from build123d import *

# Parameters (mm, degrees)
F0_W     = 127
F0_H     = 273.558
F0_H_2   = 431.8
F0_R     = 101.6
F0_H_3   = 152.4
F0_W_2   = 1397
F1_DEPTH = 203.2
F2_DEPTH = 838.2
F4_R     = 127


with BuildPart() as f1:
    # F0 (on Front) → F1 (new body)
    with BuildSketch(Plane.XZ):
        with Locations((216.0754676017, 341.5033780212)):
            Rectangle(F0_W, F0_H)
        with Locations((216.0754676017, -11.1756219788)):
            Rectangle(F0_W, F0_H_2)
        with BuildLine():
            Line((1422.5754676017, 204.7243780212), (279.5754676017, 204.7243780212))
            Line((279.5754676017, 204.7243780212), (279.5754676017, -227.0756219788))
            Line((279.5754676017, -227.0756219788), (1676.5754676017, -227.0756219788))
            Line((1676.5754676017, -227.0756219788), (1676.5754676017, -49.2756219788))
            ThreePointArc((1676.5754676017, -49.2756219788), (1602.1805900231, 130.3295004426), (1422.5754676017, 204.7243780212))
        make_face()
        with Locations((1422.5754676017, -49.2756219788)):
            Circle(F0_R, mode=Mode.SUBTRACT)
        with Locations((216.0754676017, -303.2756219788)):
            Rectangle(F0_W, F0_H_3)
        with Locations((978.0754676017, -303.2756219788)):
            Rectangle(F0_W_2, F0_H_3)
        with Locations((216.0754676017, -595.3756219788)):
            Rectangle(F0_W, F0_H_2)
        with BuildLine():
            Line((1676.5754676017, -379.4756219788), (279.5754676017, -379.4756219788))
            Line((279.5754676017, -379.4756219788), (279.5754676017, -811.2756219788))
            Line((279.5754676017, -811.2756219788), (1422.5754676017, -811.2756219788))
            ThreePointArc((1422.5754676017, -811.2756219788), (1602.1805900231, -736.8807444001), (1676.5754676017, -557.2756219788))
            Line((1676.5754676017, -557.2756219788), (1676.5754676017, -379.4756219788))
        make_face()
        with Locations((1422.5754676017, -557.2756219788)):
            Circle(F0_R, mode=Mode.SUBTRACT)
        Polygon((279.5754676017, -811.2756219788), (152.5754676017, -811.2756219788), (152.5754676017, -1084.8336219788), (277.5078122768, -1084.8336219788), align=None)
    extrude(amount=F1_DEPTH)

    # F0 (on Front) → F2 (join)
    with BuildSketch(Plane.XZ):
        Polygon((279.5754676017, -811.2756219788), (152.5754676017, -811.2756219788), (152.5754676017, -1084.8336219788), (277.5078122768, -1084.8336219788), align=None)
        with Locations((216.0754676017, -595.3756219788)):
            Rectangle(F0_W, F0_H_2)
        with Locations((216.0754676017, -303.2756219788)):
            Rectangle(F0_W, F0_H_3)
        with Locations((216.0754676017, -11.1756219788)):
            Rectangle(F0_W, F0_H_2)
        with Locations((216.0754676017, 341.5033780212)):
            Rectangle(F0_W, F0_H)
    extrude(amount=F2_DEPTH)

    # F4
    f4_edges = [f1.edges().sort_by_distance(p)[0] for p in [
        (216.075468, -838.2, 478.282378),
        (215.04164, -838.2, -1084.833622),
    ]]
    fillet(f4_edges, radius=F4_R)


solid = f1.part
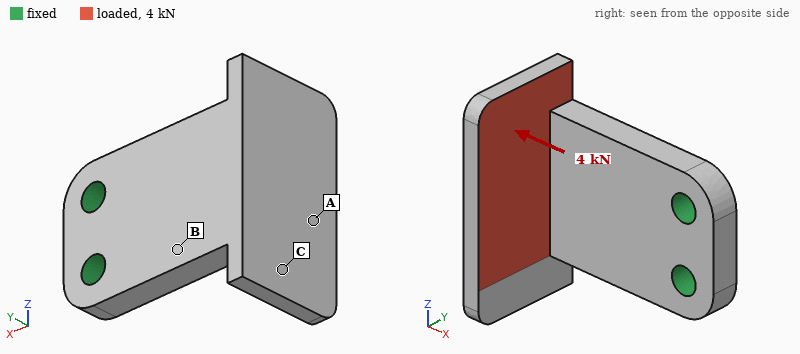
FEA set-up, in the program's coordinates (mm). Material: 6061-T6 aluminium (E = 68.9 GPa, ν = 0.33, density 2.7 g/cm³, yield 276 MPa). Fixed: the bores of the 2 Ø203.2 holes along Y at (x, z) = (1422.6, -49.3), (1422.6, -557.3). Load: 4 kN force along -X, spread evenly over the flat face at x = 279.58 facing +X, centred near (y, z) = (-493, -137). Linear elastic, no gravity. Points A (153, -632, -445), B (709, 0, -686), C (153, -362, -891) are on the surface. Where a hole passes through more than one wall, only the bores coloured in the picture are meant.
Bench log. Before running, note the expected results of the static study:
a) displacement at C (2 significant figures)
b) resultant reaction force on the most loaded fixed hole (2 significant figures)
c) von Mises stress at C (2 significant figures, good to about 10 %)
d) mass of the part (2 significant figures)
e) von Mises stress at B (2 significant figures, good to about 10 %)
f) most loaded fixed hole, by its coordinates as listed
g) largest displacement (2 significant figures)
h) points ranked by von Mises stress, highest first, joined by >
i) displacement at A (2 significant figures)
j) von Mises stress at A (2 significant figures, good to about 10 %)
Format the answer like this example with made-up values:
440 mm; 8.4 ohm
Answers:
25 µm; 3.1 kN; 0.12 MPa; 1200 kg; 0.21 MPa; (1422.6, -49.3); 47 µm; B > C > A; 34 µm; 0.057 MPa
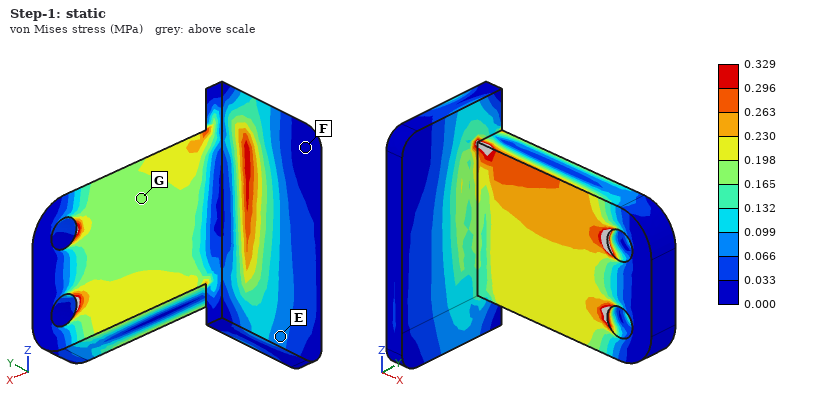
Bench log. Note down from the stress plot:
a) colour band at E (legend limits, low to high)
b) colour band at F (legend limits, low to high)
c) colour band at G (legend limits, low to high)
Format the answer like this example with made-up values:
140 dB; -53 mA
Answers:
0.066 to 0.099 MPa; 0.000 to 0.033 MPa; 0.165 to 0.198 MPa
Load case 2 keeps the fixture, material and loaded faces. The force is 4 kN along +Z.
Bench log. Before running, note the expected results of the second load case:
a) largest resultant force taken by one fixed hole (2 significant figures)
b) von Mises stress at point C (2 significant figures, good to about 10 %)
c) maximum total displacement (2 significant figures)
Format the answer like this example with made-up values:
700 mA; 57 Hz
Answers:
7.4 kN; 0.036 MPa; 25 µm
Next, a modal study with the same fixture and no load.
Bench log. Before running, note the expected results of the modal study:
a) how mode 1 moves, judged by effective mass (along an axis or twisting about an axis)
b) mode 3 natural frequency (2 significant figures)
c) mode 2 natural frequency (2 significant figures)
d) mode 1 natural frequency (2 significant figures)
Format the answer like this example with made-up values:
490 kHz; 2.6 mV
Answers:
along Y; 170 Hz; 100 Hz; 59 Hz
